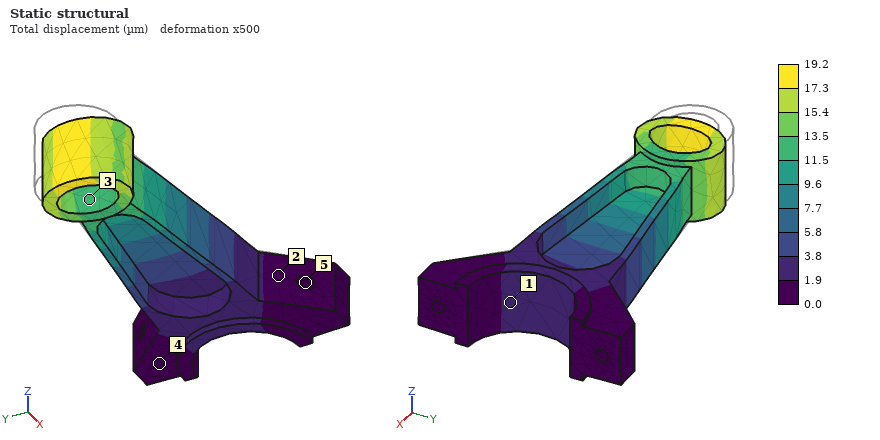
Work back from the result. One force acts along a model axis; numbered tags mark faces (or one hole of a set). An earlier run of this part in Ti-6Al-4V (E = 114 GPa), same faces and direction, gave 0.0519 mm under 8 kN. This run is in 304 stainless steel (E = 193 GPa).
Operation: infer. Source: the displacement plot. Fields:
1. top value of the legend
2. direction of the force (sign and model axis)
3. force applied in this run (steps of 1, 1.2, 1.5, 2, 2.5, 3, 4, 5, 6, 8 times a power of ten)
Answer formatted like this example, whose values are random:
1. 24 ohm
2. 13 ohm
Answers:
1. 19.2 µm
2. +X
3. 5 kN
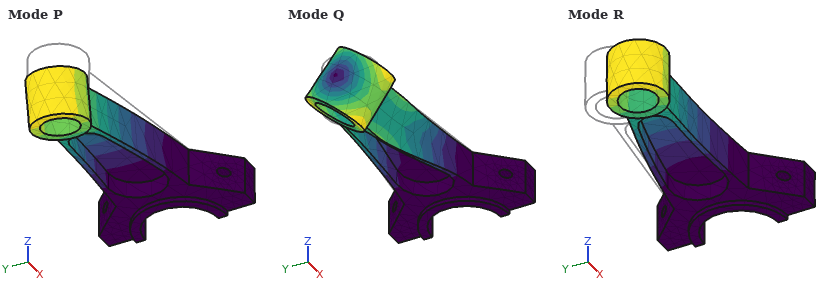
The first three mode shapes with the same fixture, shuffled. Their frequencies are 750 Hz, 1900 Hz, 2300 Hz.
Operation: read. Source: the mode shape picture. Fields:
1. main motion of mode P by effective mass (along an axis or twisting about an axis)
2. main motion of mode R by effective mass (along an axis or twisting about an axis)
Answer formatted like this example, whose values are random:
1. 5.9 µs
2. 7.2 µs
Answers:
1. along Z
2. along Y
